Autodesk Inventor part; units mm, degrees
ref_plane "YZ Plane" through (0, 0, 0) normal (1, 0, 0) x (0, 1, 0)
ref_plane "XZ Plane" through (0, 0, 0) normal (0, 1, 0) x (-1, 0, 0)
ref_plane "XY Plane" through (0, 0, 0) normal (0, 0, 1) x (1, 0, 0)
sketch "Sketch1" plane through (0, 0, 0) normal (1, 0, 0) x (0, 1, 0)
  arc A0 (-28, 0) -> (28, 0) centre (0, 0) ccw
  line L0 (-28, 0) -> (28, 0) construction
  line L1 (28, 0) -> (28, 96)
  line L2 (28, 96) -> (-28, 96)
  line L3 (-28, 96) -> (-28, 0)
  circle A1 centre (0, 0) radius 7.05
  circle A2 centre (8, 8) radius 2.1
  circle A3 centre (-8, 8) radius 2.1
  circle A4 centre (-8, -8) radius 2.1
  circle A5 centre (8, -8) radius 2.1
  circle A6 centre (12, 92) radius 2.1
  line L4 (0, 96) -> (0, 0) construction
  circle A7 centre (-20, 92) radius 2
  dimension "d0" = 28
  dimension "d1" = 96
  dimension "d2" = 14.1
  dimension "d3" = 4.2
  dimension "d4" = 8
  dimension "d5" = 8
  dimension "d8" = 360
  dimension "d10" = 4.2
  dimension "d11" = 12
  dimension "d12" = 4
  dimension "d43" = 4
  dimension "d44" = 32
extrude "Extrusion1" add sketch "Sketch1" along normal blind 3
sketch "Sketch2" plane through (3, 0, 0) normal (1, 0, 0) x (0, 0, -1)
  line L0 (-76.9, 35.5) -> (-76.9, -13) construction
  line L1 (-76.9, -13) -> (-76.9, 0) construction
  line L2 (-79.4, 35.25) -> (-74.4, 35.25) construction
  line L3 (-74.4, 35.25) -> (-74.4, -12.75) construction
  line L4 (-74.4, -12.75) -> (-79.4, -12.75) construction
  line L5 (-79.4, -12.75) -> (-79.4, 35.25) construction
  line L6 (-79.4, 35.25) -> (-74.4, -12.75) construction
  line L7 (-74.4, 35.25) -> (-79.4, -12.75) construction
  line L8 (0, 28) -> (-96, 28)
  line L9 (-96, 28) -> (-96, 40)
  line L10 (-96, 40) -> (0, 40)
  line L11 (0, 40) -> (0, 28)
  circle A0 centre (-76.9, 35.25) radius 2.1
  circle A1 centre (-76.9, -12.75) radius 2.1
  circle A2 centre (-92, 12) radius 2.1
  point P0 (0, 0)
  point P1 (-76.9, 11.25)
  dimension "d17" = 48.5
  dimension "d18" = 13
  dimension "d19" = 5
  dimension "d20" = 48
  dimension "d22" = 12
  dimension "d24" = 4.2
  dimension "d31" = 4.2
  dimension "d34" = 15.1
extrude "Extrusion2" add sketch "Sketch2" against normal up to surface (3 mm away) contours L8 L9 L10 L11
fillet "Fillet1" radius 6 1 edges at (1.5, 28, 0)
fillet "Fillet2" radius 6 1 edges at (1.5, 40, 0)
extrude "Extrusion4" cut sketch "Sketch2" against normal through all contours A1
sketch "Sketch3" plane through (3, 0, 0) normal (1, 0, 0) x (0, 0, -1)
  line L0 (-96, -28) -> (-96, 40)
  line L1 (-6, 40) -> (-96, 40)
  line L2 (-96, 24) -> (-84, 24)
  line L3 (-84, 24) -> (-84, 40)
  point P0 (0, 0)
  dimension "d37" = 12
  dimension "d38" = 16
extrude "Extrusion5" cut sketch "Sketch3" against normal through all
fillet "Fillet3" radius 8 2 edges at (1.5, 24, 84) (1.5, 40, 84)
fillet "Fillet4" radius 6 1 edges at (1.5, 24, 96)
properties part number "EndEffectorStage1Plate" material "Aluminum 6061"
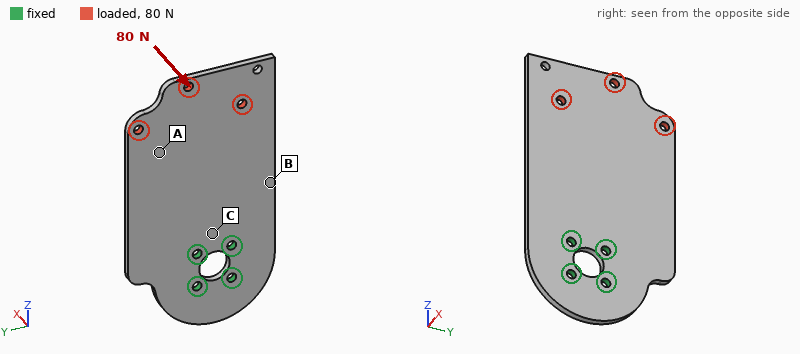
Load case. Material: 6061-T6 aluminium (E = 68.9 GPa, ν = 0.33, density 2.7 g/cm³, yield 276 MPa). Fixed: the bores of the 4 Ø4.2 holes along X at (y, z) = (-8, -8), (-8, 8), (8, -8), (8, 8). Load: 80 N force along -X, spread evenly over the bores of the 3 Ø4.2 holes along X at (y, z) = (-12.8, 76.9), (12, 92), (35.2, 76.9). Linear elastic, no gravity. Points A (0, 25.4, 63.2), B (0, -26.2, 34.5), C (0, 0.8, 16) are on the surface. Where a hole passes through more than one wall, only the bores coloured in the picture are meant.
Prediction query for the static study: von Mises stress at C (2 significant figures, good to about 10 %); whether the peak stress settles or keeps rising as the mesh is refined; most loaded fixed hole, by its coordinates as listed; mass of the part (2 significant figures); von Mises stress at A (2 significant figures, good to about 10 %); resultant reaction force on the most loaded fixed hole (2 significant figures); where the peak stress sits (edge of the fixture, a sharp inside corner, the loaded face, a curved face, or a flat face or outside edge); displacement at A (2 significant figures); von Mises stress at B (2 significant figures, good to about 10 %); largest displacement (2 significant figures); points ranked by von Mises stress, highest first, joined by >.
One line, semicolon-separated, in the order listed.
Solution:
58 MPa; keeps rising; (8, 8); 59 g; 15 MPa; 160 N; edge of the fixture; 0.72 mm; 39 MPa; 1.4 mm; C > B > A
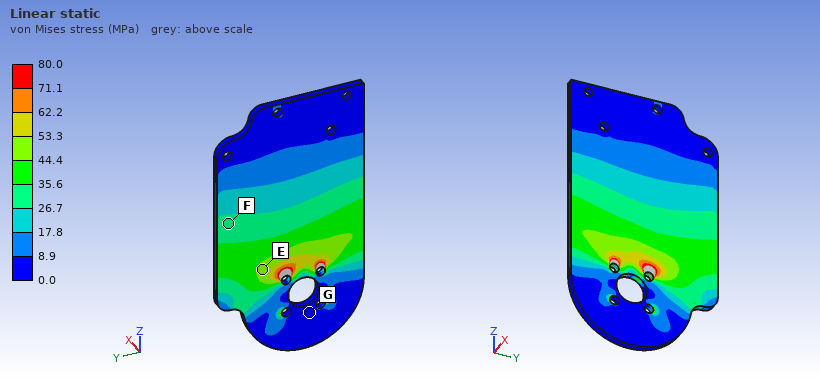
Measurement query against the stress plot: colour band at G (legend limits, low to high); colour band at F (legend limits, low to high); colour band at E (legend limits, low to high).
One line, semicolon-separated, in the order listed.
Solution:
0.0 to 8.9 MPa; 26.7 to 35.6 MPa; 44.4 to 53.3 MPa
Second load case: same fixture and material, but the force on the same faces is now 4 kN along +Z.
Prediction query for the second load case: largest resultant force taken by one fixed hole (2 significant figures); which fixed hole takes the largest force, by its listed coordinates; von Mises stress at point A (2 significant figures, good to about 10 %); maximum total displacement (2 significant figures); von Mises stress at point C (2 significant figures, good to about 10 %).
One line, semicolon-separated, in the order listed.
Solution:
2.5 kN; (8, 8); 22 MPa; 74 µm; 27 MPa
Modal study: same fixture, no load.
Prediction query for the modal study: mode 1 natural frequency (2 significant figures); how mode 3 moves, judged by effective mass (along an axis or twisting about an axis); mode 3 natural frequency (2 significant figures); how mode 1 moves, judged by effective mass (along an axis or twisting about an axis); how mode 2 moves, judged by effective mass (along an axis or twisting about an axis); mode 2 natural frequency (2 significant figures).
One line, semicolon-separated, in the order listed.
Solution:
330 Hz; along X; 1900 Hz; along X; twisting about Z; 890 Hz
